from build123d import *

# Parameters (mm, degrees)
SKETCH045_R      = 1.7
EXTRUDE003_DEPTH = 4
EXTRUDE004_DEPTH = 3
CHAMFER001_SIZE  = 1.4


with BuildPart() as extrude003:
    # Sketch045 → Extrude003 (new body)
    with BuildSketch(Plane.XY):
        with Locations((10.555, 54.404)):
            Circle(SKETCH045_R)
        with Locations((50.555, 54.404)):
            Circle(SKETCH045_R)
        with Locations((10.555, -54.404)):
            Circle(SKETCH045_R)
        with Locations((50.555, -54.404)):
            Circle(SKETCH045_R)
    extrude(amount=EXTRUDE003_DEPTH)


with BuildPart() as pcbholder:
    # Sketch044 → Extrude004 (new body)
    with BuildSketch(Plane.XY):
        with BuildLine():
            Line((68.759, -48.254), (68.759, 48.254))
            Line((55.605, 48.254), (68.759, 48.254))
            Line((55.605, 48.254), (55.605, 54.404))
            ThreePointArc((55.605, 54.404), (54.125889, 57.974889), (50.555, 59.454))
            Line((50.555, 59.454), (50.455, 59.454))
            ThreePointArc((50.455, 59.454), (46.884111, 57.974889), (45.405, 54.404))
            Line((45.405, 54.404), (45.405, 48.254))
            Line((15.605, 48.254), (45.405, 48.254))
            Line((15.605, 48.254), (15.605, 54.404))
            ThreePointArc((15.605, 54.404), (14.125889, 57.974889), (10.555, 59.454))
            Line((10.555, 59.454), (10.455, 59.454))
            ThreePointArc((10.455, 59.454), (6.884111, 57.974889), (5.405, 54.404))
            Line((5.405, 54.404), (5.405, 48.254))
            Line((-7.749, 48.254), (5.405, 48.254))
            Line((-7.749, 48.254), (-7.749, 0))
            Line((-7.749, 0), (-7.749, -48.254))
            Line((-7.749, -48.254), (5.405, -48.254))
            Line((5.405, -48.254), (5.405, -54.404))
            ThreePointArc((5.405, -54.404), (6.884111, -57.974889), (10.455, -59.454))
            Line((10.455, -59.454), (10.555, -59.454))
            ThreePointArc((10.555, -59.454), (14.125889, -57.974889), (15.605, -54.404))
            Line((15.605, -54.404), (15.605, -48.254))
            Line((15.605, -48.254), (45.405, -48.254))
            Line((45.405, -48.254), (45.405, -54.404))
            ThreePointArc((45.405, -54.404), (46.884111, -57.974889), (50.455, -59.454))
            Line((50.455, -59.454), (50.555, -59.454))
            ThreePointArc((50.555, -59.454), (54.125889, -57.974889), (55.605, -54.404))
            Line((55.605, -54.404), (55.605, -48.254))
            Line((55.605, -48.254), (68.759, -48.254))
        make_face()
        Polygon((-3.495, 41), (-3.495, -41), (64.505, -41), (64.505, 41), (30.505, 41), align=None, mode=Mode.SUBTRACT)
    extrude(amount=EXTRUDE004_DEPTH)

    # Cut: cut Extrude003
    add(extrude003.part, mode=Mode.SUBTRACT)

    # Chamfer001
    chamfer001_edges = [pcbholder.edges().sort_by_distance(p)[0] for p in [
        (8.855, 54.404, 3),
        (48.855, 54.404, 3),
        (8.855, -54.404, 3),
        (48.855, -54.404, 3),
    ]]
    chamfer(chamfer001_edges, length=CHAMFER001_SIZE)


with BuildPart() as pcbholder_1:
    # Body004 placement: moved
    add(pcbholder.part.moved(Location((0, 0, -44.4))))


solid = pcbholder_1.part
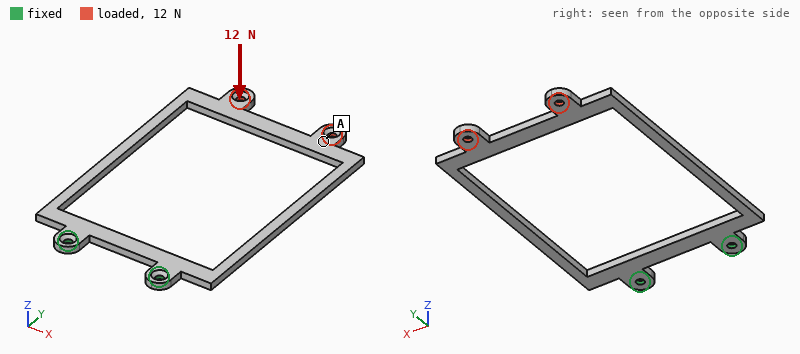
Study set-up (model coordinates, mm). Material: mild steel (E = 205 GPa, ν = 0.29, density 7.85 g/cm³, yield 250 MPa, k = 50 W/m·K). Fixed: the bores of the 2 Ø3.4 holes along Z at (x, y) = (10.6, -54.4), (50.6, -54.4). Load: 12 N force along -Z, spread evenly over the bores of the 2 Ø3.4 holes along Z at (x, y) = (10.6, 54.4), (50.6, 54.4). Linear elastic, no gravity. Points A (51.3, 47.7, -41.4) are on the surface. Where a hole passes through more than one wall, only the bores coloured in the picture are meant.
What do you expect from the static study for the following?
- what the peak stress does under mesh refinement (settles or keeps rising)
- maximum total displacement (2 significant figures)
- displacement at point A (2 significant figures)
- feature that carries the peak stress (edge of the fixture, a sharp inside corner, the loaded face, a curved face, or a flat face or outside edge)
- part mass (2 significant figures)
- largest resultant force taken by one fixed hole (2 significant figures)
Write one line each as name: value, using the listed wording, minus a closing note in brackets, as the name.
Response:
what the peak stress does under mesh refinement: keeps rising
maximum total displacement: 1.4 mm
displacement at point A: 1.2 mm
feature that carries the peak stress: edge of the fixture
part mass: 51 g
largest resultant force taken by one fixed hole: 6.0 N
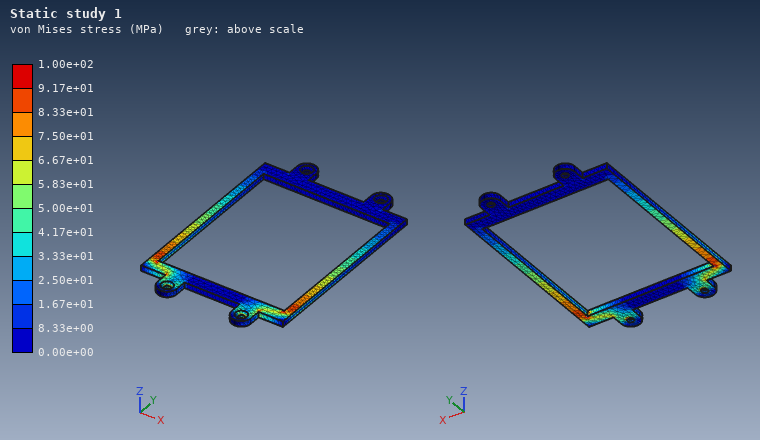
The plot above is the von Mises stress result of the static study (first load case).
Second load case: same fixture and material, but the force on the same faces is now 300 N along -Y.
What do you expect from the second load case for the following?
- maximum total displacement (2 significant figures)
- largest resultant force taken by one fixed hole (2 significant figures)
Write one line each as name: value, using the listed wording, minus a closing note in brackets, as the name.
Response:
maximum total displacement: 0.34 mm
largest resultant force taken by one fixed hole: 250 N
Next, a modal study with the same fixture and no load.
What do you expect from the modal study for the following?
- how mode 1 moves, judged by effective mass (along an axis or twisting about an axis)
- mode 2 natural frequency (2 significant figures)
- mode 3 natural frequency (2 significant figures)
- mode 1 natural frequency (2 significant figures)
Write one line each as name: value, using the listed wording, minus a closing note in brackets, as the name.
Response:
how mode 1 moves, judged by effective mass: along Z
mode 2 natural frequency: 350 Hz
mode 3 natural frequency: 350 Hz
mode 1 natural frequency: 120 Hz
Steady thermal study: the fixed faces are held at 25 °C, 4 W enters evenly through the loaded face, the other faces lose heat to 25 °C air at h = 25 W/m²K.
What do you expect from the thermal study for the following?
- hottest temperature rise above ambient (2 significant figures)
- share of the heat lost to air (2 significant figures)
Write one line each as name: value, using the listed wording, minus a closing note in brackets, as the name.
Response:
hottest temperature rise above ambient: 65 K
share of the heat lost to air: 94 %
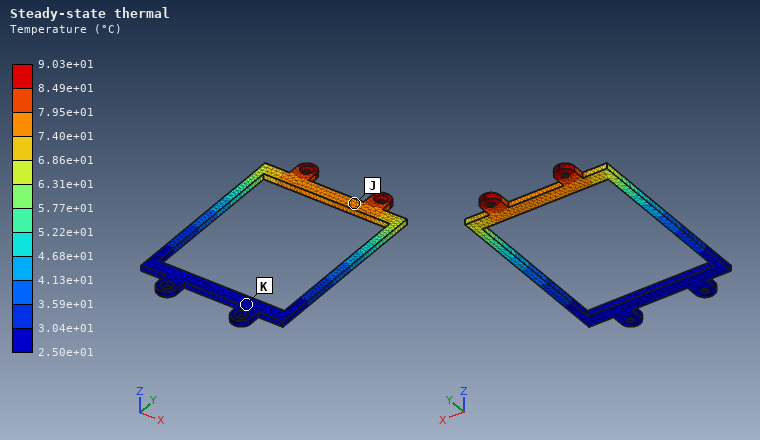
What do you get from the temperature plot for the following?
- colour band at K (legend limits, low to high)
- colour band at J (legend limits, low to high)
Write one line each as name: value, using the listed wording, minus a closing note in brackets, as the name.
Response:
colour band at K: 2.50e+01 to 3.04e+01 °C
colour band at J: 7.40e+01 to 7.95e+01 °C
